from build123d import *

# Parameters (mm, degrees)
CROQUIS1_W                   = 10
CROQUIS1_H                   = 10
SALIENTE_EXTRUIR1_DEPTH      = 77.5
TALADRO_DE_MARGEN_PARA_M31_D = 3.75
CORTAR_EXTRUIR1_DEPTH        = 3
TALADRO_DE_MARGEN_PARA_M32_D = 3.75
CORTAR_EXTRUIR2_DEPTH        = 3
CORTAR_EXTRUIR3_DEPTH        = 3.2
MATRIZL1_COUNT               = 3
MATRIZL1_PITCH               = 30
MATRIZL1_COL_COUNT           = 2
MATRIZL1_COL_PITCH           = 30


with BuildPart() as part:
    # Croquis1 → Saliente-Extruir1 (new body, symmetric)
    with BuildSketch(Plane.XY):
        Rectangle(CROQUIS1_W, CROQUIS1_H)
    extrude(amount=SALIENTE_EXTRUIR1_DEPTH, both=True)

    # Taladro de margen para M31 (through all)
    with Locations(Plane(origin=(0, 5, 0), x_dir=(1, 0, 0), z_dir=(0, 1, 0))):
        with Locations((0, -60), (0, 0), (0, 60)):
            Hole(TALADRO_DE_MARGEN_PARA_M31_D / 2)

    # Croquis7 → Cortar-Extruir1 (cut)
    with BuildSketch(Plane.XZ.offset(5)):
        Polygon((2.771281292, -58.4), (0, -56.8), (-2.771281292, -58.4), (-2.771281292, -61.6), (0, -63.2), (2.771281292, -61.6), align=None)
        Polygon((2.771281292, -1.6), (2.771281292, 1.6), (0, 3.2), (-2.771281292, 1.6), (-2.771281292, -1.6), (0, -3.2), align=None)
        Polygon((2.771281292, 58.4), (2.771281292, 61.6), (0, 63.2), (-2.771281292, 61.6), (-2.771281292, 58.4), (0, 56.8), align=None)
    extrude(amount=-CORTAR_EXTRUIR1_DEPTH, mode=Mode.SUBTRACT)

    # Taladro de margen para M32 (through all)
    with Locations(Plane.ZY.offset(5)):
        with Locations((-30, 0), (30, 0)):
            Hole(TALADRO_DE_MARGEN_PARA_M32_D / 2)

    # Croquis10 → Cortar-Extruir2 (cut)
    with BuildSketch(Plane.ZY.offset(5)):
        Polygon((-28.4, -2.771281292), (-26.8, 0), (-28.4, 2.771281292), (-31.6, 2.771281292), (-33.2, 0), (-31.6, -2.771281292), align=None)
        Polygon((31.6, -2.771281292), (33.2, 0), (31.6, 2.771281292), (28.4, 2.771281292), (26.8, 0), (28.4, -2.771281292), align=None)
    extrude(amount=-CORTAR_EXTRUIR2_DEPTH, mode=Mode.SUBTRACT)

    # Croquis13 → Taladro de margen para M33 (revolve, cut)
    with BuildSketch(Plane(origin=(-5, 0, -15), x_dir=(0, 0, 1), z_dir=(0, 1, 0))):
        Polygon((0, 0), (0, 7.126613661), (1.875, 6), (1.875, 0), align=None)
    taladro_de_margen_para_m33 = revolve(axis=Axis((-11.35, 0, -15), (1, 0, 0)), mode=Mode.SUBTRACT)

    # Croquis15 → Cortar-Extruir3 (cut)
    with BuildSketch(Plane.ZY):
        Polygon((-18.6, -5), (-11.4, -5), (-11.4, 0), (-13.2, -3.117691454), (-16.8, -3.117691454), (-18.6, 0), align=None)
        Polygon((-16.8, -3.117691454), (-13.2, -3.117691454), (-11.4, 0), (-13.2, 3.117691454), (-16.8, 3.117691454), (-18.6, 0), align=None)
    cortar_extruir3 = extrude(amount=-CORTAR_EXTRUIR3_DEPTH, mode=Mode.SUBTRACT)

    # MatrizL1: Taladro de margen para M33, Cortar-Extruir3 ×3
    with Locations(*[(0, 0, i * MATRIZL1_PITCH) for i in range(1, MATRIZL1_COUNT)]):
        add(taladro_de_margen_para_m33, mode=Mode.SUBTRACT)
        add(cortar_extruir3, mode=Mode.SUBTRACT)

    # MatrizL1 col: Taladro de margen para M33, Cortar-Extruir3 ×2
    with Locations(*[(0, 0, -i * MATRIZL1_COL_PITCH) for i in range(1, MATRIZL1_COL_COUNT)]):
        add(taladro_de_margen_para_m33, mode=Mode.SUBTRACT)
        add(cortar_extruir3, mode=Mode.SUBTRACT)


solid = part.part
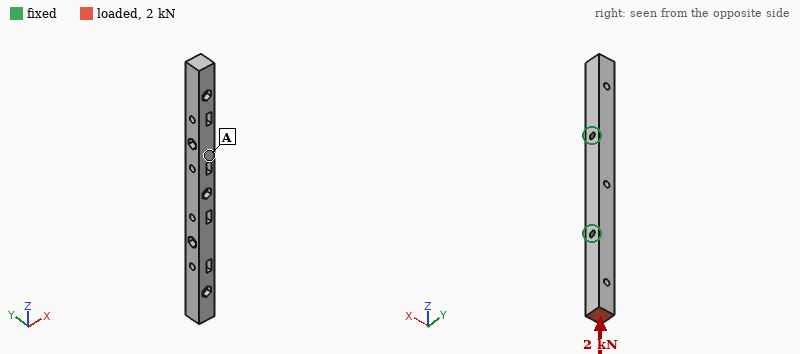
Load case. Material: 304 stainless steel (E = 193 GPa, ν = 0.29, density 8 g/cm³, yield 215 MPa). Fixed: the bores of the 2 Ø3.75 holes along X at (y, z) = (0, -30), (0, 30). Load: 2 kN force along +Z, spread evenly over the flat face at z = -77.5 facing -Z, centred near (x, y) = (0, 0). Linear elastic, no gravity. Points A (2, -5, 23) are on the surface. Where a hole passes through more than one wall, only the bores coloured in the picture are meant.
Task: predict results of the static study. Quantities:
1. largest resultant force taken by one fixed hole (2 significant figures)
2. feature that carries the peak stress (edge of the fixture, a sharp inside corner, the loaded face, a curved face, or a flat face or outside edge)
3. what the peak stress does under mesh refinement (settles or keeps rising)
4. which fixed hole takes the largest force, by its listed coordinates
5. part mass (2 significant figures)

1.9 kN
edge of the fixture
keeps rising
(0, -30)
110 g
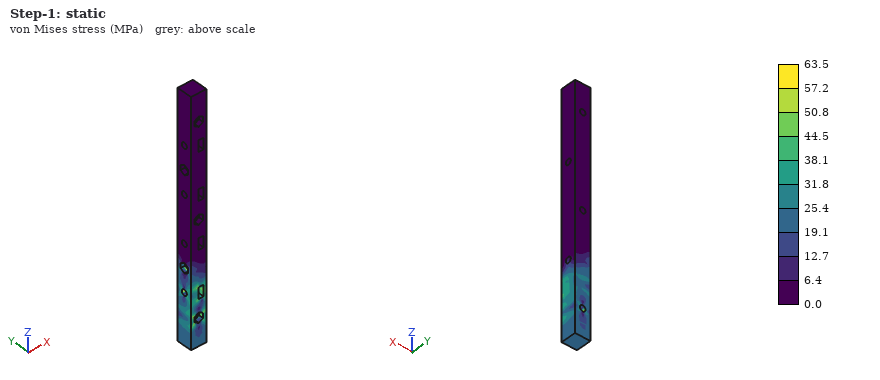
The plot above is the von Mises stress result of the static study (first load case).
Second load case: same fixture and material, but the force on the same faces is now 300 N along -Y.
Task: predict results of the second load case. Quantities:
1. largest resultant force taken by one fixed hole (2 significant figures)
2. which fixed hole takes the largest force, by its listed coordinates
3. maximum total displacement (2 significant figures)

370 N
(0, -30)
98 µm
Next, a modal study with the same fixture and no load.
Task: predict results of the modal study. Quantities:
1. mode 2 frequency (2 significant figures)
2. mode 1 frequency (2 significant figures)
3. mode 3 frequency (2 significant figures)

2900 Hz
2800 Hz
3000 Hz
